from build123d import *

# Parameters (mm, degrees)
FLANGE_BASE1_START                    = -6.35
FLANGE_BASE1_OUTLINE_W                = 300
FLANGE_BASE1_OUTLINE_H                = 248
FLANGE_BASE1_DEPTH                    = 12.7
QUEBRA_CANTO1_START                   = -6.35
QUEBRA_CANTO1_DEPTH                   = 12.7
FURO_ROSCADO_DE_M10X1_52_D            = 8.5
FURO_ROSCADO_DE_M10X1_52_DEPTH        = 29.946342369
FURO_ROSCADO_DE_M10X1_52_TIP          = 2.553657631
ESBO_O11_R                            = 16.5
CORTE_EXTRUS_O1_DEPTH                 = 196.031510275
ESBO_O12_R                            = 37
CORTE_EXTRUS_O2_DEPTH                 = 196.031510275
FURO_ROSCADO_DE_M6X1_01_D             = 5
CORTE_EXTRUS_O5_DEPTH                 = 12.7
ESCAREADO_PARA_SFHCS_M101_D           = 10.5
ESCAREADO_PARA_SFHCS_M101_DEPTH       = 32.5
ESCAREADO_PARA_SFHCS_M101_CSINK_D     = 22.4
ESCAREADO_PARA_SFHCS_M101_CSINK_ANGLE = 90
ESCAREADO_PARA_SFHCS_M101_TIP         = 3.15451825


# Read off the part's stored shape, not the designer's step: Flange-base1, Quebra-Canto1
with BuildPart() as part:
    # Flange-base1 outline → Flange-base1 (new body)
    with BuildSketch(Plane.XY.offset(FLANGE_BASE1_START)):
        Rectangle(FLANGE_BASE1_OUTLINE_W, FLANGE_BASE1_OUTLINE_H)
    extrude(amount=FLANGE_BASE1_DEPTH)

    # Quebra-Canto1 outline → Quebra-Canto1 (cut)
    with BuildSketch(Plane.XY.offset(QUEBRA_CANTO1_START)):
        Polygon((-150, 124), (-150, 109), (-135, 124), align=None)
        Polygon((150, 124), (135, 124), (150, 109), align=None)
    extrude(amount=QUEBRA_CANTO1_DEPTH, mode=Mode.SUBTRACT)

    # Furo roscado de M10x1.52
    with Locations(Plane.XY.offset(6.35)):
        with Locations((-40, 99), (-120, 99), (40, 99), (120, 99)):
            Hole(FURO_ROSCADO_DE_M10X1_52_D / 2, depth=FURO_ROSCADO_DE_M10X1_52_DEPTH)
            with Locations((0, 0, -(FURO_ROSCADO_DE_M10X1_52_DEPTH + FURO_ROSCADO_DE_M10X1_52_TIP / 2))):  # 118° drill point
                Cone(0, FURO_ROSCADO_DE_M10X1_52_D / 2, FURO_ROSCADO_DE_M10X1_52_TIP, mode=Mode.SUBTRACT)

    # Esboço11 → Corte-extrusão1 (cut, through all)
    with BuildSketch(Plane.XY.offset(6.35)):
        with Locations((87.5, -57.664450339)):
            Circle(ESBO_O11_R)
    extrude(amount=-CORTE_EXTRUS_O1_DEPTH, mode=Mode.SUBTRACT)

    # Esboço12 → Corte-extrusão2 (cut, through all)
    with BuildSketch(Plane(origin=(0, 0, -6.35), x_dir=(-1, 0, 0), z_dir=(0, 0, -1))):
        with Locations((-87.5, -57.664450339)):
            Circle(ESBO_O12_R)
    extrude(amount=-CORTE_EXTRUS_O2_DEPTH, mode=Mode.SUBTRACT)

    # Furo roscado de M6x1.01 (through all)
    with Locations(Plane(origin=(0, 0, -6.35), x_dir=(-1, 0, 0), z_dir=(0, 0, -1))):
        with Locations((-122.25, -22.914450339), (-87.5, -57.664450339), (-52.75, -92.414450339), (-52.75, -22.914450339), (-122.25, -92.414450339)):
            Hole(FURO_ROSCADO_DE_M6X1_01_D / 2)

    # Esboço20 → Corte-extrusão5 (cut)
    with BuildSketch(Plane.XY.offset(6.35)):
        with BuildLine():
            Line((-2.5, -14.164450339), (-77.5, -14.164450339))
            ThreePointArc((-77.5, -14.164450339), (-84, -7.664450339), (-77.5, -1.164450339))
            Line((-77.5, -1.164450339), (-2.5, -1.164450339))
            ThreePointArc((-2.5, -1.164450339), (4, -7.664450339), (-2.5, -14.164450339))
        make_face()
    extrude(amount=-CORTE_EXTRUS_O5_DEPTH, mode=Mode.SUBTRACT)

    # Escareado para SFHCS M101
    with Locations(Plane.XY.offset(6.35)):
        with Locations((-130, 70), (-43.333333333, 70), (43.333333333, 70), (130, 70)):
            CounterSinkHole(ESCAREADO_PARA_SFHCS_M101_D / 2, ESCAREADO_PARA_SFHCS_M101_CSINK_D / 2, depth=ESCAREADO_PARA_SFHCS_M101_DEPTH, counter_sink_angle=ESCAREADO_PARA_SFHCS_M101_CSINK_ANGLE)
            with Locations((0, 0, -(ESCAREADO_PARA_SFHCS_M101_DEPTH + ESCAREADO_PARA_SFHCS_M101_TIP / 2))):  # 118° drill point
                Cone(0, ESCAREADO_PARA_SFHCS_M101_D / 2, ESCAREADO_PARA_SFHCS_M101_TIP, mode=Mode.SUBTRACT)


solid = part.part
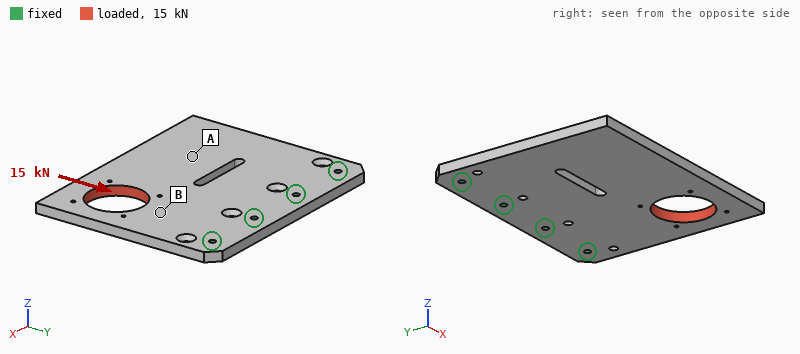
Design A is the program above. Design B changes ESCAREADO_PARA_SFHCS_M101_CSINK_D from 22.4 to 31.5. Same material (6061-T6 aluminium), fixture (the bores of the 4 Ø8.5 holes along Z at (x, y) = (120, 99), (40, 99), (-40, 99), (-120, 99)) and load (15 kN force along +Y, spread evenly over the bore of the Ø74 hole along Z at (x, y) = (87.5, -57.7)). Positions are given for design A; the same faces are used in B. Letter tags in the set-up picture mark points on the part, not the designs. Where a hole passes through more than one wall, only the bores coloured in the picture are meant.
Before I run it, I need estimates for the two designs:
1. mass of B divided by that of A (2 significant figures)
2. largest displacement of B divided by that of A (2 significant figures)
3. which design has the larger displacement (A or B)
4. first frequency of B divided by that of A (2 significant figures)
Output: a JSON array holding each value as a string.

["0.99", "1.2", "B", "0.97"]
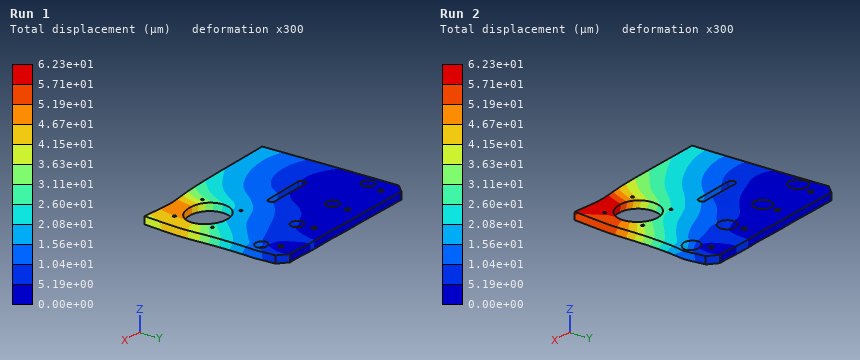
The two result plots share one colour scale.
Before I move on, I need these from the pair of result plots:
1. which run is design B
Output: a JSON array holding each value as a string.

["Run 2"]
